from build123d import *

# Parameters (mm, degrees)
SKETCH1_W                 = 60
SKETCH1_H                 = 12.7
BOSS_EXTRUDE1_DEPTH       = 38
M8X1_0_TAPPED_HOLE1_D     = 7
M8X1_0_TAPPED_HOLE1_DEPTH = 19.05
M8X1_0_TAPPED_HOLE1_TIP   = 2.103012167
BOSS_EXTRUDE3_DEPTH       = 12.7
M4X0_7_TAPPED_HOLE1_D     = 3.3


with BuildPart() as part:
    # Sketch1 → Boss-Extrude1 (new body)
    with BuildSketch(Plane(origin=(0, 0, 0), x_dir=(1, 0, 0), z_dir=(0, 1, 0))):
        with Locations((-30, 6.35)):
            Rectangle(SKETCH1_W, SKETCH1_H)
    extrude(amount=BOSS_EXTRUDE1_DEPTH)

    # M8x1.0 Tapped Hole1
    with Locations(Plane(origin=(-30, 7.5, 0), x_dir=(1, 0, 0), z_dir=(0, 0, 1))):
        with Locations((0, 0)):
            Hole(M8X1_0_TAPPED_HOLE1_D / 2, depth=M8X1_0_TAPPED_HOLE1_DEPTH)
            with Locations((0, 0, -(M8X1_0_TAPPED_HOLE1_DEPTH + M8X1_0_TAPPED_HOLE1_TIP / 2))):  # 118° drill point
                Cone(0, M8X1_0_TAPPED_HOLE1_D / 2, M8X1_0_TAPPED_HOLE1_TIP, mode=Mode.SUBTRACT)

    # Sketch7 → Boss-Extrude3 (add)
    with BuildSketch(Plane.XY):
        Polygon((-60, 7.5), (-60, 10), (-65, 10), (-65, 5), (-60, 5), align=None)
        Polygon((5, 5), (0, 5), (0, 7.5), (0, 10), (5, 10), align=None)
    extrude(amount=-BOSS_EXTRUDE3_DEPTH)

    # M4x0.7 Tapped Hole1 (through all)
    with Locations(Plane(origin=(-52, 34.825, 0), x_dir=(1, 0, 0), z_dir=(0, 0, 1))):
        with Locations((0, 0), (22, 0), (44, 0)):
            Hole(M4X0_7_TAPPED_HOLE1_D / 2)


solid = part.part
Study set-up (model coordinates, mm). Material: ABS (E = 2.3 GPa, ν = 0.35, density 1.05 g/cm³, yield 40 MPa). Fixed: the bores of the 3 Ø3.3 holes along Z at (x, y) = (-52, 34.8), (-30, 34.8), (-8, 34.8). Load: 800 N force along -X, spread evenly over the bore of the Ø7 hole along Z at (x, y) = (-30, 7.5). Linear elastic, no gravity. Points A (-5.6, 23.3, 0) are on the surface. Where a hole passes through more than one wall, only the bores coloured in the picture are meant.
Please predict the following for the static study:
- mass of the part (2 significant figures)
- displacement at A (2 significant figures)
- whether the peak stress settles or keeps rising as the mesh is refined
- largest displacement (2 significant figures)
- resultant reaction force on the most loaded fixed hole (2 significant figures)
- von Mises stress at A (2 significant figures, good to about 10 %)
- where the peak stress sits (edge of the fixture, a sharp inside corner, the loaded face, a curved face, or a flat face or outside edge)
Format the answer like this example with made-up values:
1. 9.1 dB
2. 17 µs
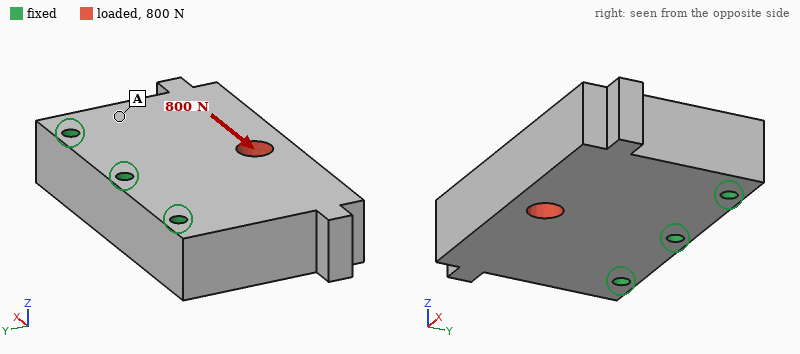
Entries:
1. 30 g
2. 30 µm
3. keeps rising
4. 75 µm
5. 520 N
6. 1.7 MPa
7. edge of the fixture
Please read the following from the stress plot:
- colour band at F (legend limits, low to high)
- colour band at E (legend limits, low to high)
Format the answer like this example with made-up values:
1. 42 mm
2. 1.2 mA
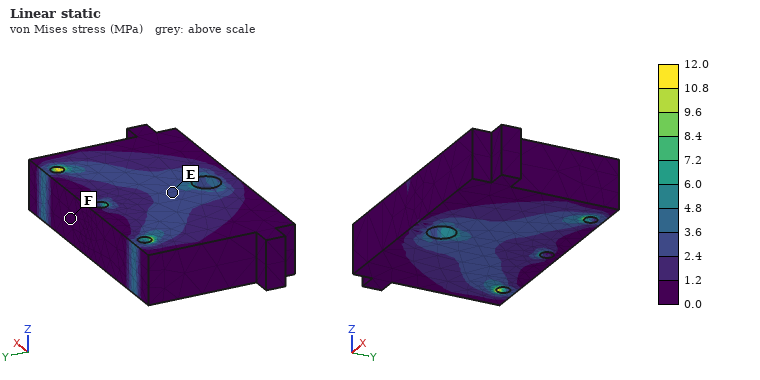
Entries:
1. 0.0 to 1.2 MPa
2. 2.4 to 3.6 MPa
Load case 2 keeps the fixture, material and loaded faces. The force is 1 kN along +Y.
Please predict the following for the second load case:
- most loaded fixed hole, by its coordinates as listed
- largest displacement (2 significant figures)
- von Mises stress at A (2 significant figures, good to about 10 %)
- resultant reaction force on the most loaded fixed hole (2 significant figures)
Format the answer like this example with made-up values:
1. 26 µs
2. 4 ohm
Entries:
1. (-30, 34.8)
2. 59 µm
3. 0.74 MPa
4. 470 N
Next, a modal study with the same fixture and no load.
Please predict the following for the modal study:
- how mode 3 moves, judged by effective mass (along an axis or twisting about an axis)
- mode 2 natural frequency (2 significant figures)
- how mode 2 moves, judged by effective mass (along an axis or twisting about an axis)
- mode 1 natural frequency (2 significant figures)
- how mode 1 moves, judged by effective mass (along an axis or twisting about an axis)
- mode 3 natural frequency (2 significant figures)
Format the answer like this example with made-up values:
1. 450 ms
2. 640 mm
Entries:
1. along X
2. 2900 Hz
3. twisting about Y
4. 1900 Hz
5. along Z
6. 4500 Hz
